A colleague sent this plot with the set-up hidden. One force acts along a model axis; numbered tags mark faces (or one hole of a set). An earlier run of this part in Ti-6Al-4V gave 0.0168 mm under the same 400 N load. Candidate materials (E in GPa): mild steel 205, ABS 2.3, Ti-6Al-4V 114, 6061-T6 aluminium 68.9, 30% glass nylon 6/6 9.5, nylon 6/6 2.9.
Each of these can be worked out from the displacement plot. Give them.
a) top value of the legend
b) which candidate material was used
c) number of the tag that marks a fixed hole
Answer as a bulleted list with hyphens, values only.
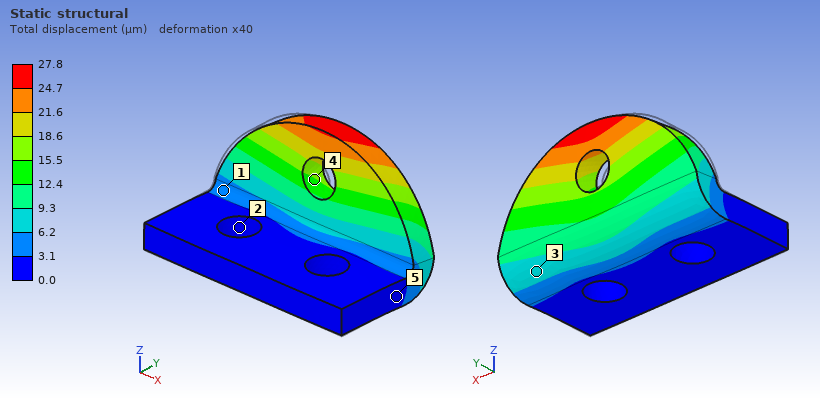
- 27.8 µm
- 6061-T6 aluminium
- 2
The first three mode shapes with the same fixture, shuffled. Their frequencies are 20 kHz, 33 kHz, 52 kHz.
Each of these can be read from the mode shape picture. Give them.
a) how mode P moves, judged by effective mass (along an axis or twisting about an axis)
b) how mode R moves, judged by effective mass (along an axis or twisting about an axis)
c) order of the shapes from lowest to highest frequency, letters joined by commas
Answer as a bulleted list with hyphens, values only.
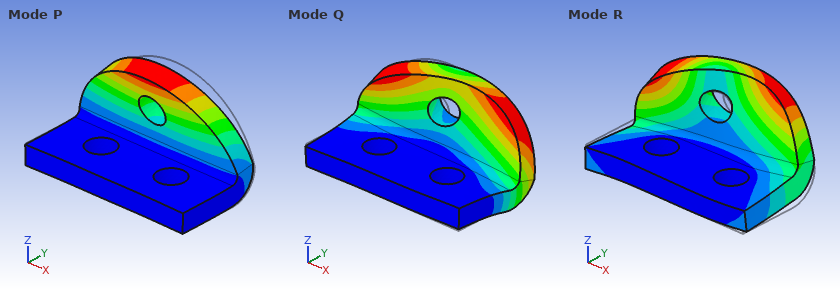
- along Y
- along X
- P, Q, R
